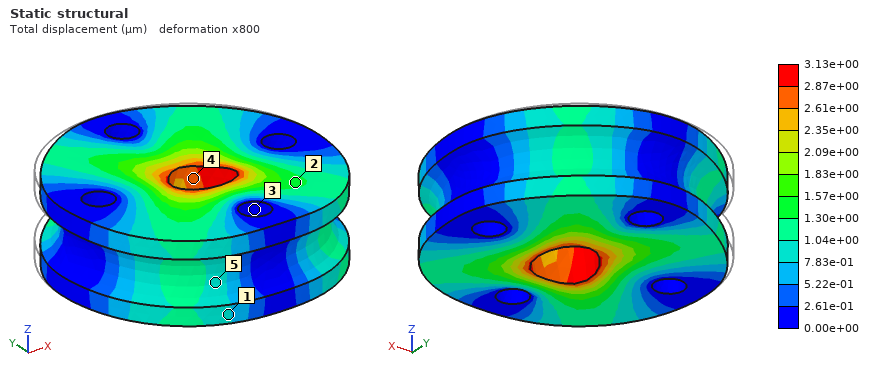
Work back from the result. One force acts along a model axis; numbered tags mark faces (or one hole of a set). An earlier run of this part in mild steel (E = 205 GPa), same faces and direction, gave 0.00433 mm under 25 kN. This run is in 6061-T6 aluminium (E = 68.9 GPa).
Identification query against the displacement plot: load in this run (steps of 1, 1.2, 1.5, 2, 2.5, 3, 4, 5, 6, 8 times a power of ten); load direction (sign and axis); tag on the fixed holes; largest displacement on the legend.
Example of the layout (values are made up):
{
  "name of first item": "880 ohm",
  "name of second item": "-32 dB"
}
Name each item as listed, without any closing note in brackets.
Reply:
{
  "load in this run": "6 kN",
  "load direction": "-Y",
  "tag on the fixed holes": "3",
  "largest displacement on the legend": "3.13e+00 µm"
}
